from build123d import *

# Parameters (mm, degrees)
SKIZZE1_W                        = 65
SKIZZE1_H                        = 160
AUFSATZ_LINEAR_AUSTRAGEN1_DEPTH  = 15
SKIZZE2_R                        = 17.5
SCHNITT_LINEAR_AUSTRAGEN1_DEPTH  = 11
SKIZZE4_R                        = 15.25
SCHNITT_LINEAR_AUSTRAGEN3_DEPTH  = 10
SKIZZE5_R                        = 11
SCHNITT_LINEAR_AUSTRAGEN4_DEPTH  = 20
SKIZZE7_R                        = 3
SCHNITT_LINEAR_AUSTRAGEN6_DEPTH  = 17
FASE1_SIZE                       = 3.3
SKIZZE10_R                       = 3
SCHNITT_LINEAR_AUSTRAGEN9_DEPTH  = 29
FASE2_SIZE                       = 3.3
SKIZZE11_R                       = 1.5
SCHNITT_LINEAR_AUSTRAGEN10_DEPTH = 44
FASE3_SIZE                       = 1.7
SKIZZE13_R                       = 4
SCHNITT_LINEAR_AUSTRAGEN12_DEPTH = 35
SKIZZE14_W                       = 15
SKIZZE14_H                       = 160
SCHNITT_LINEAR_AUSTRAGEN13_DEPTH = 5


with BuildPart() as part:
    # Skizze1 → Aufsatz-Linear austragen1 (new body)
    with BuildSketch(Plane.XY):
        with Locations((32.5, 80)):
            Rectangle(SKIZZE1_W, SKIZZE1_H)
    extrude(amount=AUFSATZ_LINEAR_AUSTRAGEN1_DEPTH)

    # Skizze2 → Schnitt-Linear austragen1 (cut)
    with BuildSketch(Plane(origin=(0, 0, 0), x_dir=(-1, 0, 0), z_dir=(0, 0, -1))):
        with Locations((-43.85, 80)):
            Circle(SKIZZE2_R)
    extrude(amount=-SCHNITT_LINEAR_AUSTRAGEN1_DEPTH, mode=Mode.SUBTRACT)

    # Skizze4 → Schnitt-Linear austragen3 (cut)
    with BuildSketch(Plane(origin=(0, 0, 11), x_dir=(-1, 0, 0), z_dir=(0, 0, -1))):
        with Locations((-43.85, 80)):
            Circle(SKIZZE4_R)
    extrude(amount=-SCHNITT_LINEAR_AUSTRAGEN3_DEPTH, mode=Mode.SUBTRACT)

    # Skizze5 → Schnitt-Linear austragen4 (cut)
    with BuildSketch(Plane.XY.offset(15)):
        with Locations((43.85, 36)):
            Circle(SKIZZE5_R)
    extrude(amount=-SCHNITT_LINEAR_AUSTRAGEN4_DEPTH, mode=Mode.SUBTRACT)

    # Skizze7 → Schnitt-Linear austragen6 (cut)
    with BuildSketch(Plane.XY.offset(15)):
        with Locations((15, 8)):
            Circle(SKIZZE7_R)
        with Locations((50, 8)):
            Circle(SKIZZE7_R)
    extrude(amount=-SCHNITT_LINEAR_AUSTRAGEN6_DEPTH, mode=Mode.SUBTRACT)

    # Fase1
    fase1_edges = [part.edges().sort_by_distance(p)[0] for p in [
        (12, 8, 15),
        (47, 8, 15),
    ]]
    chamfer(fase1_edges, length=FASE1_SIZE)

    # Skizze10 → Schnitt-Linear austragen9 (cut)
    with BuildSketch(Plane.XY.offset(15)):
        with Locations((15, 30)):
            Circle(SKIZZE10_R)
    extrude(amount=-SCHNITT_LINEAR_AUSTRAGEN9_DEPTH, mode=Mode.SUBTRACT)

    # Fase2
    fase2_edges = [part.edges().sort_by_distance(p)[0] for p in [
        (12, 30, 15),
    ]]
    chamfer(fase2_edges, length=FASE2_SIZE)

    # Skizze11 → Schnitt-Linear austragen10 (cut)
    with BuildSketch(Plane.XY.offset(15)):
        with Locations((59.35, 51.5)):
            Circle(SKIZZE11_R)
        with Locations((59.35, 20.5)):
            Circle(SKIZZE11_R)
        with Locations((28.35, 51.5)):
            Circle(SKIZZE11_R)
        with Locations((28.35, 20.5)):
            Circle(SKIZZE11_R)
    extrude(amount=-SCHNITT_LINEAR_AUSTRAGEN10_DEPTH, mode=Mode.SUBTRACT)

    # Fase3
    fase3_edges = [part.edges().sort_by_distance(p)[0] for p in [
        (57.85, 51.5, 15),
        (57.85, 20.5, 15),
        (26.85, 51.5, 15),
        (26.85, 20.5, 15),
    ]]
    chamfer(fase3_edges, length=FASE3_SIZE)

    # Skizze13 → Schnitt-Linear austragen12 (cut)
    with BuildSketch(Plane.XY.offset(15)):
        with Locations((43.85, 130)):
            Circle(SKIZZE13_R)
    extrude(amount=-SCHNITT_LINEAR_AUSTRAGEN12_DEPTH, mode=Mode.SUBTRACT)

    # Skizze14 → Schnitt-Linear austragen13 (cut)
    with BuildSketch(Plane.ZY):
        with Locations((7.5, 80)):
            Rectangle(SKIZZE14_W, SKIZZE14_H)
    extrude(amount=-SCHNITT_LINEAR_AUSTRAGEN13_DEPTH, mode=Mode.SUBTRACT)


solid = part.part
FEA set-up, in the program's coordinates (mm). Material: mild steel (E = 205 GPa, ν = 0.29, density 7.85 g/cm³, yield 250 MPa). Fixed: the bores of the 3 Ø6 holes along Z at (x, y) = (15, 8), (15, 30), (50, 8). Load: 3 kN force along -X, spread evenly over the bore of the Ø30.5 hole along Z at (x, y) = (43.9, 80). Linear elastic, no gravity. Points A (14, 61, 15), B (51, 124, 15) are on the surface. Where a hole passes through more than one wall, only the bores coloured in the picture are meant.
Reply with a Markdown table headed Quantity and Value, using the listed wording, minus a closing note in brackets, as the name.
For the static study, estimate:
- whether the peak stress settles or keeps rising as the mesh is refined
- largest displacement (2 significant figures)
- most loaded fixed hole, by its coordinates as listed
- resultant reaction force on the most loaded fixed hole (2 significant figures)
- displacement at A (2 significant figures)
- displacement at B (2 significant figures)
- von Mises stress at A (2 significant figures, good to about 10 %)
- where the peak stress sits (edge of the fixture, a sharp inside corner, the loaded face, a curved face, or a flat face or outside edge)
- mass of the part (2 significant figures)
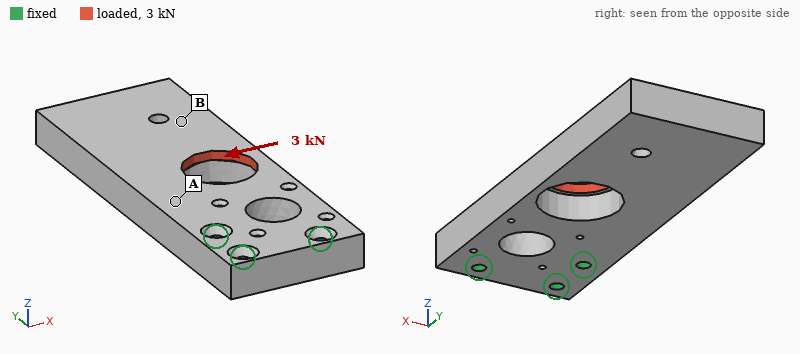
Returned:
| Quantity | Value |
|---|---|
| whether the peak stress settles or keeps rising as the mesh is refined | keeps rising |
| largest displacement | 34 µm |
| most loaded fixed hole, by its coordinates as listed | (15, 30) |
| resultant reaction force on the most loaded fixed hole | 4.6 kN |
| displacement at A | 8.2 µm |
| displacement at B | 26 µm |
| von Mises stress at A | 12 MPa |
| where the peak stress sits | edge of the fixture |
| mass of the part | 960 g |
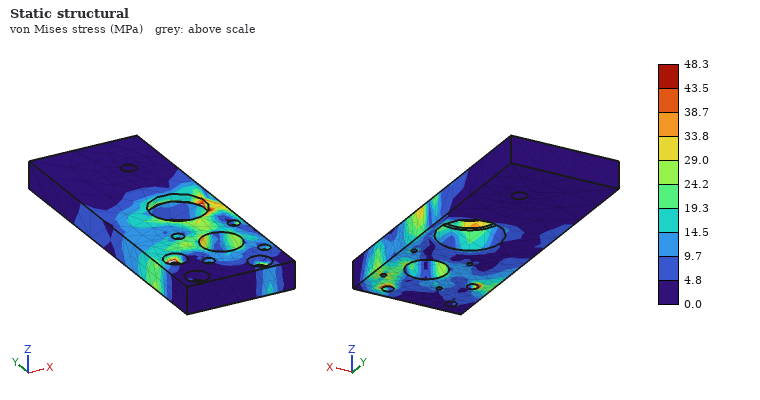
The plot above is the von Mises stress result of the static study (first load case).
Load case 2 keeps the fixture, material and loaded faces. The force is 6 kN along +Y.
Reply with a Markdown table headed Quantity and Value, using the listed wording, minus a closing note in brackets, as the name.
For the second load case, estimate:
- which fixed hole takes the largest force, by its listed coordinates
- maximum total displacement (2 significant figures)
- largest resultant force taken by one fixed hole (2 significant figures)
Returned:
| Quantity | Value |
|---|---|
| which fixed hole takes the largest force, by its listed coordinates | (50, 8) |
| maximum total displacement | 0.10 mm |
| largest resultant force taken by one fixed hole | 4.1 kN |
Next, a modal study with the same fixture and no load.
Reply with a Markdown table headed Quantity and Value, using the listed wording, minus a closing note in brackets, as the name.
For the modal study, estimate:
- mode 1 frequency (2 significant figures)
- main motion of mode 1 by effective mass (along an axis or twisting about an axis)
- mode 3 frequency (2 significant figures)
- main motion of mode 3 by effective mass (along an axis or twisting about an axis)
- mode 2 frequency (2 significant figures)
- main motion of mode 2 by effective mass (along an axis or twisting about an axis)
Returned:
| Quantity | Value |
|---|---|
| mode 1 frequency | 530 Hz |
| main motion of mode 1 by effective mass | along Z |
| mode 3 frequency | 2200 Hz |
| main motion of mode 3 by effective mass | twisting about Y |
| mode 2 frequency | 1700 Hz |
| main motion of mode 2 by effective mass | along X |
